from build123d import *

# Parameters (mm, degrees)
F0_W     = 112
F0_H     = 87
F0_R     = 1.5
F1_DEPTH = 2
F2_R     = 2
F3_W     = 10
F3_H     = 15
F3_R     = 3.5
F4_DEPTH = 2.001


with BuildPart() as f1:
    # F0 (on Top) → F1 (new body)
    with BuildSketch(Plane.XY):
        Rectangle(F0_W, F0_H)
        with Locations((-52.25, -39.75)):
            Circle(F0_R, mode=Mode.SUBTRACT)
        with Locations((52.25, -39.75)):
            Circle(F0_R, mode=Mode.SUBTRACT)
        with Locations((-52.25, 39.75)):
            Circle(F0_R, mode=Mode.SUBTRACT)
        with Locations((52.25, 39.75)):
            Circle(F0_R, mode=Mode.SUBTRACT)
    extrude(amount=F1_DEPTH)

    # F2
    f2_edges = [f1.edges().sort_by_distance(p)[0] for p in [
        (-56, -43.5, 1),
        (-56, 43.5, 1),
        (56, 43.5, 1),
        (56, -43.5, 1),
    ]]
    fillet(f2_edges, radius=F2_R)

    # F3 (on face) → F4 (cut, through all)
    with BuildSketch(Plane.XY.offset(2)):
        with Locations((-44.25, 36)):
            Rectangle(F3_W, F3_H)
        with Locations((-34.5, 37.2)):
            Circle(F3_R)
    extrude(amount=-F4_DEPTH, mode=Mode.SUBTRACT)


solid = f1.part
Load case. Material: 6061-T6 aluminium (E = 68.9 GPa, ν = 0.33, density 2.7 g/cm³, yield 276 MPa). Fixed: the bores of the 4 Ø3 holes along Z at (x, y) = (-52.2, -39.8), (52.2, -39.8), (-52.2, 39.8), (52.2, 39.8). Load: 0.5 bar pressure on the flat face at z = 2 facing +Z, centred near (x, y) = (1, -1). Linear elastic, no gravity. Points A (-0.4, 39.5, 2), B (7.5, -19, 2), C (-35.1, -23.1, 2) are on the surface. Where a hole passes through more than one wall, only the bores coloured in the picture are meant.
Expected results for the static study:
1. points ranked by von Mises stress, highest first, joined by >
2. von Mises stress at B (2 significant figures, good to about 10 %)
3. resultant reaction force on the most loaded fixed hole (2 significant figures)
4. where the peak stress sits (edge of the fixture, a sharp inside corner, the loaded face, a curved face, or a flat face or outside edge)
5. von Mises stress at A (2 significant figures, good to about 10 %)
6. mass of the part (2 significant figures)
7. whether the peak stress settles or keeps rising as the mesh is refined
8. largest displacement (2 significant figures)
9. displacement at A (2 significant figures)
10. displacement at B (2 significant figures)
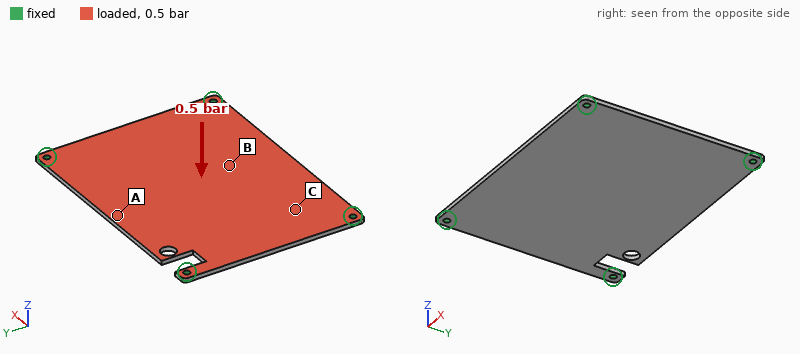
A > B > C
42 MPa
130 N
edge of the fixture
59 MPa
51 g
keeps rising
0.85 mm
0.82 mm
0.68 mm
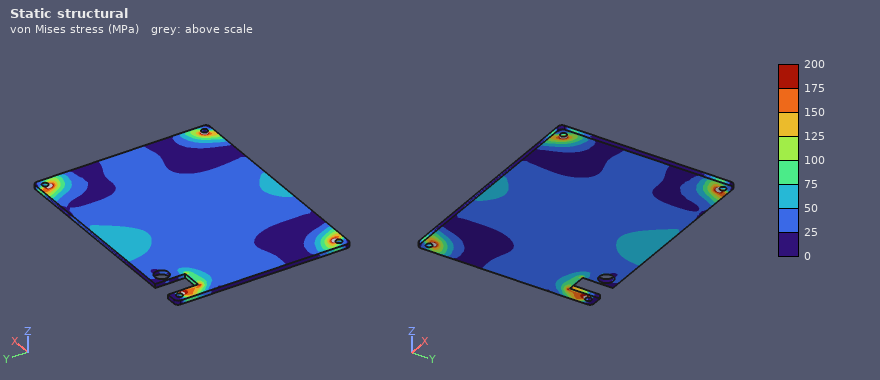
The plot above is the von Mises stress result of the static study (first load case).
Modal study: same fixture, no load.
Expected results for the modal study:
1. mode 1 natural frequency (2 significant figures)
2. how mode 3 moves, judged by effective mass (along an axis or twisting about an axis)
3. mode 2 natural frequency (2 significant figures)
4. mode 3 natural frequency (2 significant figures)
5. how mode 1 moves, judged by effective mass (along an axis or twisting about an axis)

620 Hz
twisting about Y
1000 Hz
1500 Hz
along Z
